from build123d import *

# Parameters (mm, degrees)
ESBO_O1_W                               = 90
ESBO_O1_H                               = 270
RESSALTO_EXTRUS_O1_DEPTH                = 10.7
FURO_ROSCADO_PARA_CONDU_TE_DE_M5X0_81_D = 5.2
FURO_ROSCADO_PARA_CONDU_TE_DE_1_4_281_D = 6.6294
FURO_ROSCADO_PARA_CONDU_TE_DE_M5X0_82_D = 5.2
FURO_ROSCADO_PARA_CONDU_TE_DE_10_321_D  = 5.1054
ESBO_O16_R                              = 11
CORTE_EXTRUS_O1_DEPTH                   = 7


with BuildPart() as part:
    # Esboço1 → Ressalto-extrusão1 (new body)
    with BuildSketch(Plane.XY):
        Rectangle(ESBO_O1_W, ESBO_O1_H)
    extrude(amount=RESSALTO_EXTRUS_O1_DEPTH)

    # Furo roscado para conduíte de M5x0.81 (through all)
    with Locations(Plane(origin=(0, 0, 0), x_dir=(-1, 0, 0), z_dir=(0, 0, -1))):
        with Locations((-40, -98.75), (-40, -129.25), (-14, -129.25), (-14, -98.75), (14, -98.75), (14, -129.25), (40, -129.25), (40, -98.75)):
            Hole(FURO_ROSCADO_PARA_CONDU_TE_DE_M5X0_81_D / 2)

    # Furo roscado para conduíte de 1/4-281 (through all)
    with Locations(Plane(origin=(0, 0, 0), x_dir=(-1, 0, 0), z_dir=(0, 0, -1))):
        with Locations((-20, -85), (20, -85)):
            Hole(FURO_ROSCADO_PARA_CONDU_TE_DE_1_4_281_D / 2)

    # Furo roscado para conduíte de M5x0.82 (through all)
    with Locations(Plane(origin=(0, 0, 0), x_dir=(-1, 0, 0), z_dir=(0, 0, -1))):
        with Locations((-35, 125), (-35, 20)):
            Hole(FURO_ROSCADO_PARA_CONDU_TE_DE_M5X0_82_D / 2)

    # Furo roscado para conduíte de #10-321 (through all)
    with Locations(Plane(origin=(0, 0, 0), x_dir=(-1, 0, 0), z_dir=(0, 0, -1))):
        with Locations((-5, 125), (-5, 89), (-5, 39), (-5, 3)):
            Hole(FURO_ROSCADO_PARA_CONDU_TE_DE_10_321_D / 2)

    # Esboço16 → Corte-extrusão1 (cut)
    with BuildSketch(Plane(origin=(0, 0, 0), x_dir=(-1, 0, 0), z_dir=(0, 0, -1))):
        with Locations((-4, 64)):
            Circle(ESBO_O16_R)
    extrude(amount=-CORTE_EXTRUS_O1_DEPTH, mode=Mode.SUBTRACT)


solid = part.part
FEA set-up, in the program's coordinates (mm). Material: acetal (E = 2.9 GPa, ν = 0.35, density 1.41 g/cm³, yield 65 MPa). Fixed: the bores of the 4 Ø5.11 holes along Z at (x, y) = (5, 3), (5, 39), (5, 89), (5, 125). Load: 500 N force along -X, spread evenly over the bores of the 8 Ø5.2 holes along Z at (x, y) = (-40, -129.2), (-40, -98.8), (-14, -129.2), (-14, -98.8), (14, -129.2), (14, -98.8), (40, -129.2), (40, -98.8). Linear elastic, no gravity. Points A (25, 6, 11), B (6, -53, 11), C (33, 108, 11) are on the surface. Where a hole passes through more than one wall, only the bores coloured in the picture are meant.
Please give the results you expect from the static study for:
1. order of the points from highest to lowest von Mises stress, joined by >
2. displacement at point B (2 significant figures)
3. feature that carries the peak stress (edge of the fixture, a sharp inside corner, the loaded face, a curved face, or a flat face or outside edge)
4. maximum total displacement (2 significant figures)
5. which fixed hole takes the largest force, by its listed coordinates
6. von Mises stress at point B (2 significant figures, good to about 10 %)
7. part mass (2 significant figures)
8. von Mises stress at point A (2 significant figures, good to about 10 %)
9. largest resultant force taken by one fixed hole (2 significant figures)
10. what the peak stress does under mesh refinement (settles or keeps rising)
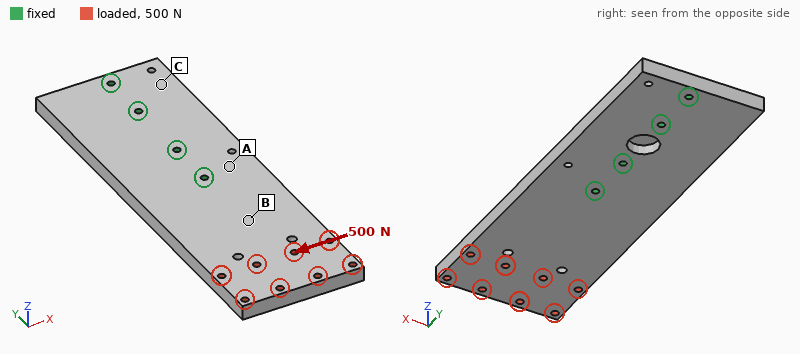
A > B > C
0.19 mm
edge of the fixture
0.55 mm
(5, 3)
1.3 MPa
360 g
2.7 MPa
1.2 kN
keeps rising
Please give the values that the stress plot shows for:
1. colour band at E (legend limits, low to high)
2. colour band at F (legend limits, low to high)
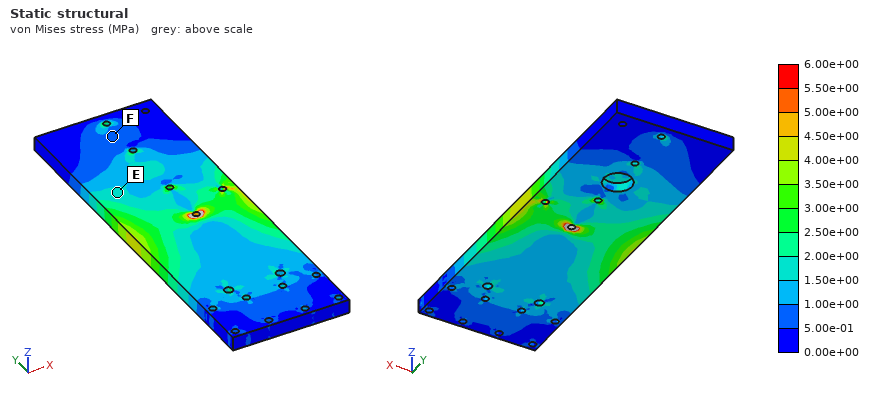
1.50e+00 to 2.00e+00 MPa
5.00e-01 to 1.00e+00 MPa
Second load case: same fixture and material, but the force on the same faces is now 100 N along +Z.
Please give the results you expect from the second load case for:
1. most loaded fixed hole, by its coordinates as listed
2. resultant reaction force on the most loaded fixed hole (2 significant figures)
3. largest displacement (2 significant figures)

(5, 3)
290 N
3.0 mm
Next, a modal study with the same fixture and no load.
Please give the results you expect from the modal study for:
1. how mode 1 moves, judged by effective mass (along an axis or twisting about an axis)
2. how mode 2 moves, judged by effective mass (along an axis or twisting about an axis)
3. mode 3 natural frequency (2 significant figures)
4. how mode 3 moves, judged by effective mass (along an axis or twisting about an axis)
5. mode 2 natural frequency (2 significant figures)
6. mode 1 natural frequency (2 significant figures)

along Z
twisting about Y
580 Hz
along X
330 Hz
120 Hz
